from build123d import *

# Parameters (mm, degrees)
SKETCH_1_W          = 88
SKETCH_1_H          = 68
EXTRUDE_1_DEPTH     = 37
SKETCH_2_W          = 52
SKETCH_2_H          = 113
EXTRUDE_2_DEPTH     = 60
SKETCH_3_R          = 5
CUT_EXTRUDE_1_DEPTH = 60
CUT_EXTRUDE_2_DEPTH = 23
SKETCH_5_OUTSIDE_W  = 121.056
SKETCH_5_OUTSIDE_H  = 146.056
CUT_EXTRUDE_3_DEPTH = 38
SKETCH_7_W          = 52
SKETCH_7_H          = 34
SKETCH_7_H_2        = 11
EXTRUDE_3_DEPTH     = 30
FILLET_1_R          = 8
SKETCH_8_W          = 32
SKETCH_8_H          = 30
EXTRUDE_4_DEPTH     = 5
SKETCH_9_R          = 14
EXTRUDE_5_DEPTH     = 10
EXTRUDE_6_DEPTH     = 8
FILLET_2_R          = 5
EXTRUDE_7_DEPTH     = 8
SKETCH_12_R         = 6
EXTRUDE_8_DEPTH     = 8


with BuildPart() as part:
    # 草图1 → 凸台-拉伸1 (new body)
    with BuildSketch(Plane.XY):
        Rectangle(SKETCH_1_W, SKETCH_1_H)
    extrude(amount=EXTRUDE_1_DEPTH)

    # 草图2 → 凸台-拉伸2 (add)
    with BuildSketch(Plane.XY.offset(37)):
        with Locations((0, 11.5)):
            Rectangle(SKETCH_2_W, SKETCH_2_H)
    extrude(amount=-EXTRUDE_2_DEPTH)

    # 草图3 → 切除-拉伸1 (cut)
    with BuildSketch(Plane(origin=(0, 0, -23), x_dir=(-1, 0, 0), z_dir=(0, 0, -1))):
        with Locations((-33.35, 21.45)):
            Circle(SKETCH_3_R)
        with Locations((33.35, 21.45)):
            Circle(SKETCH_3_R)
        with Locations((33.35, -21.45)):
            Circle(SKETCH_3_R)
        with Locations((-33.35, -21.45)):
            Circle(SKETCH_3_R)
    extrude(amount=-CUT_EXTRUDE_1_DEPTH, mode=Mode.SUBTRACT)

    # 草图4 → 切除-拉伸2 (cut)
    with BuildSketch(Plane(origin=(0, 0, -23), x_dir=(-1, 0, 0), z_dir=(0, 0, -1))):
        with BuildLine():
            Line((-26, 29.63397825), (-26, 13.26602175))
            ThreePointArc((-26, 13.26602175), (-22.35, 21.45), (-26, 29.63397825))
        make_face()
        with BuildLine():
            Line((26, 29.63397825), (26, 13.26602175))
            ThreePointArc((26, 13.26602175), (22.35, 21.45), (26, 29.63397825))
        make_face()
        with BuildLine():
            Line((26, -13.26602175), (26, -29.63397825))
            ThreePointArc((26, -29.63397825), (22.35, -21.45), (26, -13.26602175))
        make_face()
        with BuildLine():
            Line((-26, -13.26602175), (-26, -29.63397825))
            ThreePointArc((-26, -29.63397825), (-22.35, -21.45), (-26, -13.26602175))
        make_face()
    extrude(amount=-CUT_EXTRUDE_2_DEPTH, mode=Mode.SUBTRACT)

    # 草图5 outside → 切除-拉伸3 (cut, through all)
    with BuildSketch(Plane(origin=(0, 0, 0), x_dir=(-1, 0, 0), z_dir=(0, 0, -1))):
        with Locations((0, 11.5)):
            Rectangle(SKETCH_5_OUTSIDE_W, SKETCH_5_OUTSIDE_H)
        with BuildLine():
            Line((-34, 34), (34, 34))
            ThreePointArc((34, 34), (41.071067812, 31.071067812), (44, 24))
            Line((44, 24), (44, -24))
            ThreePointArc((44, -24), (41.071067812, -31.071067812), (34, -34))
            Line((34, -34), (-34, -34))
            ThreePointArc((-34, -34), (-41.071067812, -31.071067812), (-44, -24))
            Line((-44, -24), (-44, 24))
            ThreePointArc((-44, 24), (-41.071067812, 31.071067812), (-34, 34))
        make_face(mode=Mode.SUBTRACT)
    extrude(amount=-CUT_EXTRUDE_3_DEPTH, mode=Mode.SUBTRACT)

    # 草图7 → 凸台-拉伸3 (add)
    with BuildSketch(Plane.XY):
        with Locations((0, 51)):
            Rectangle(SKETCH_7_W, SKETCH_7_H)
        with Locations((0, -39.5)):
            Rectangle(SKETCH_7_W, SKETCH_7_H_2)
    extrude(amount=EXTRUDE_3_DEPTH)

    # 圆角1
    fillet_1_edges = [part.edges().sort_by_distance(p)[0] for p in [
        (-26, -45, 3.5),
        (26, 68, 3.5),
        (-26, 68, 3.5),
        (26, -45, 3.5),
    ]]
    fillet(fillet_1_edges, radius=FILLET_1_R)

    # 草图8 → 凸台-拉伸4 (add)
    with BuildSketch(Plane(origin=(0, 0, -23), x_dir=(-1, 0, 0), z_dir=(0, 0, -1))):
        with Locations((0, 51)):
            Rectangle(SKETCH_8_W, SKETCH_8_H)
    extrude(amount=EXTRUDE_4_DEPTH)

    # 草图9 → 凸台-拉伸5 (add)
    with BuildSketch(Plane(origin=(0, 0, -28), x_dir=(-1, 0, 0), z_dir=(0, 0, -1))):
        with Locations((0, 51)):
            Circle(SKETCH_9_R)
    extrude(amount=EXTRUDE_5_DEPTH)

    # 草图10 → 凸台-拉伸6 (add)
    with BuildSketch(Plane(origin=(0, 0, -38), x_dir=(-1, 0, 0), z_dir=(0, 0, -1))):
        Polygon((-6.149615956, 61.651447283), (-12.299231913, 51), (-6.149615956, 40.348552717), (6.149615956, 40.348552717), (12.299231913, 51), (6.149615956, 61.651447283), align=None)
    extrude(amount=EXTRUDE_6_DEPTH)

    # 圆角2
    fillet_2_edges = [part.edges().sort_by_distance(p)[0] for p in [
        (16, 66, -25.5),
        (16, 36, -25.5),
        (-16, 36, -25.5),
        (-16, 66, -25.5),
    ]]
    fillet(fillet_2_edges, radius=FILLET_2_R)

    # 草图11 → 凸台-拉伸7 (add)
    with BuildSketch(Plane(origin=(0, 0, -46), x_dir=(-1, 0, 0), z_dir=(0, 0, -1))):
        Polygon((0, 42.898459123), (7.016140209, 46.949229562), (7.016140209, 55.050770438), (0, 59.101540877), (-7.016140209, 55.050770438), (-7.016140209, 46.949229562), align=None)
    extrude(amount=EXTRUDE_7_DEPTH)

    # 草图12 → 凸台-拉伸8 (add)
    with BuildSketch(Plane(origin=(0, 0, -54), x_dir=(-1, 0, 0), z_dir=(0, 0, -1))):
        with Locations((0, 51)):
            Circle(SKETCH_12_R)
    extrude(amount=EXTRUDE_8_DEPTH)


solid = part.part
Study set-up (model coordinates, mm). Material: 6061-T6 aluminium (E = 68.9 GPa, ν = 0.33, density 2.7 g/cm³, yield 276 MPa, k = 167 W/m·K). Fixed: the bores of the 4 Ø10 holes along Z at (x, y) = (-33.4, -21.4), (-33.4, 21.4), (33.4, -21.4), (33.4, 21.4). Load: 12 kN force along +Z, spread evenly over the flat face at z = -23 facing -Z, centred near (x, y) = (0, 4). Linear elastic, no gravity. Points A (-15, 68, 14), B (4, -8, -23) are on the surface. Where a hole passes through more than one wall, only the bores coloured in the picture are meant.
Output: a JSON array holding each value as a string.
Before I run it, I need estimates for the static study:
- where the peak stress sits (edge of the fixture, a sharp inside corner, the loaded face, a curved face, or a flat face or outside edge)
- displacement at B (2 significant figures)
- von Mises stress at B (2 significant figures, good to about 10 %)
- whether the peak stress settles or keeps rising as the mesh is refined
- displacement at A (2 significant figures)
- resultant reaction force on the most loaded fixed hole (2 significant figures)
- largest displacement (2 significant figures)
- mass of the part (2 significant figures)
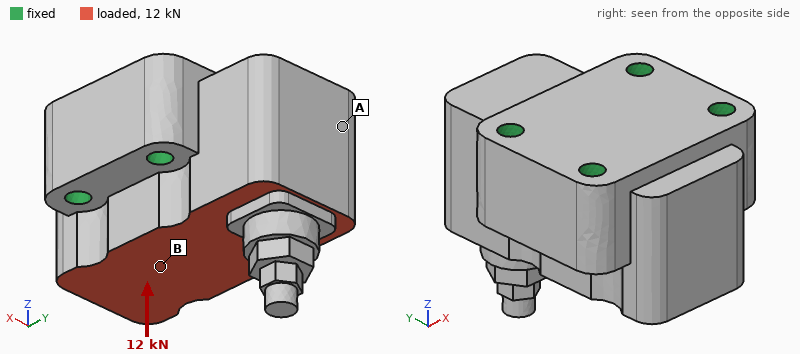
["edge of the fixture", "2.6 µm", "3.2 MPa", "keeps rising", "4.8 µm", "3.5 kN", "5.9 µm", "1.1 kg"]
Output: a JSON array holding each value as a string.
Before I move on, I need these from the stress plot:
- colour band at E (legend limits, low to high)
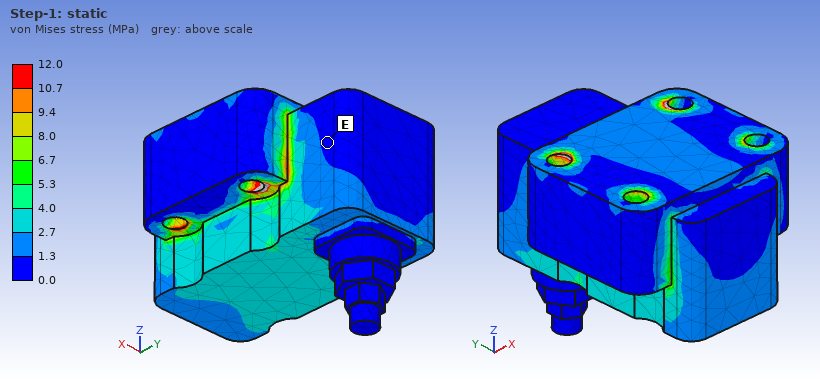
["0.0 to 1.3 MPa"]
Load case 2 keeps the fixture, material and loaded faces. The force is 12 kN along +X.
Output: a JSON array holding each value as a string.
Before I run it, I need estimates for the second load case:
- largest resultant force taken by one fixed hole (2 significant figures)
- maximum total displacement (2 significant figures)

["4.8 kN", "12 µm"]
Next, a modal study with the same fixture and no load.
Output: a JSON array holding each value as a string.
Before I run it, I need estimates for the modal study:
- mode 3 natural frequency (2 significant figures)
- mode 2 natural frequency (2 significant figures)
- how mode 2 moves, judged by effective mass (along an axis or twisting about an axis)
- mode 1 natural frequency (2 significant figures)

["13 kHz", "8700 Hz", "along X", "6200 Hz"]
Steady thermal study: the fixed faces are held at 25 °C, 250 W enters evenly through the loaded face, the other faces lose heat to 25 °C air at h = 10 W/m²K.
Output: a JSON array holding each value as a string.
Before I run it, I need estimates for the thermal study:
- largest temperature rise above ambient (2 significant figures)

["15 K"]
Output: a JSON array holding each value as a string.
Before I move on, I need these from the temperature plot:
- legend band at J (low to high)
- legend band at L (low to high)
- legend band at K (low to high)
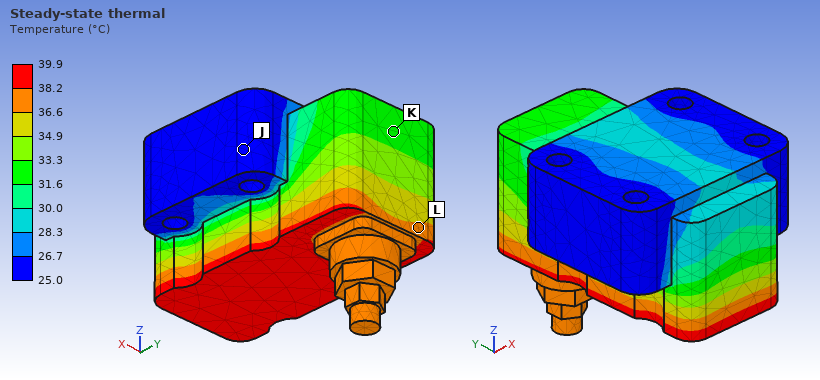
["25.0 to 26.7 °C", "36.6 to 38.2 °C", "31.6 to 33.3 °C"]
